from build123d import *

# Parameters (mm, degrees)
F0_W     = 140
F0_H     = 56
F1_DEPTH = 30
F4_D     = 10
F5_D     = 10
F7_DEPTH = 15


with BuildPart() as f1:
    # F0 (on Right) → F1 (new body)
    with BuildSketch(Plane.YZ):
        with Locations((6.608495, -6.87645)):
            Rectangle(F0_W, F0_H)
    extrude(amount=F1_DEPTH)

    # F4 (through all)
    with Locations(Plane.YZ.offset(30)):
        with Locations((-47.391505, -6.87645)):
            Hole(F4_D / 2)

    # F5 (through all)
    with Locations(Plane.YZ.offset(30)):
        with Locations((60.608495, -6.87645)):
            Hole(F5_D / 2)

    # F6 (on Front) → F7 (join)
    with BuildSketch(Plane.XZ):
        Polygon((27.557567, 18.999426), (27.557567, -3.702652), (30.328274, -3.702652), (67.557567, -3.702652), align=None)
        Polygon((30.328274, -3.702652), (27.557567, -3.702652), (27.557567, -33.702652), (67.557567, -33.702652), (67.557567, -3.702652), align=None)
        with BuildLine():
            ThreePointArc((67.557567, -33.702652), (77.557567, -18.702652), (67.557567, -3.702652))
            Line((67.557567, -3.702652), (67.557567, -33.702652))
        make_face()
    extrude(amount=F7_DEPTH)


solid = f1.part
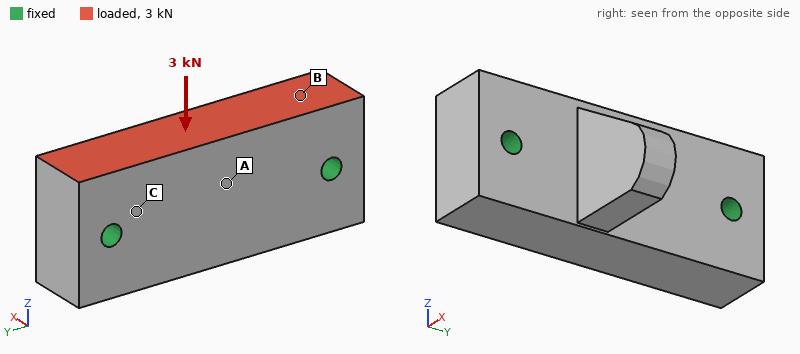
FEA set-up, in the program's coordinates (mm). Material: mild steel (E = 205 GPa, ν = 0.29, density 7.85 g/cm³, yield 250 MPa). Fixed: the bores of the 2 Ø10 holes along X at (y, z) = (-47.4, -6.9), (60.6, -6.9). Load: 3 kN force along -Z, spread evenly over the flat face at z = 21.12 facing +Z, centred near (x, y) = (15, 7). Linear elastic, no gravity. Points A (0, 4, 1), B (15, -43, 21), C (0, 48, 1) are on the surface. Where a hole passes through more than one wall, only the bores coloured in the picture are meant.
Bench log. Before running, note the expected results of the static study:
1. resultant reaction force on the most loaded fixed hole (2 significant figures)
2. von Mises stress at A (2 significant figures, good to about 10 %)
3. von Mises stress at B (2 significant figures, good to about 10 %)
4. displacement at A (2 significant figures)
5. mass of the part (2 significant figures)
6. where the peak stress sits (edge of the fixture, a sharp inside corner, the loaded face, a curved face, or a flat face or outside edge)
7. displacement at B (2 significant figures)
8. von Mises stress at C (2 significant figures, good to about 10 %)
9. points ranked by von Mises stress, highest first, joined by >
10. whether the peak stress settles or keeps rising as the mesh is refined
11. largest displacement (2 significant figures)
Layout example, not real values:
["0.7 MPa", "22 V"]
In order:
["1.5 kN", "0.48 MPa", "0.91 MPa", "0.54 µm", "2.0 kg", "edge of the fixture", "0.26 µm", "1.5 MPa", "C > B > A", "keeps rising", "0.59 µm"]
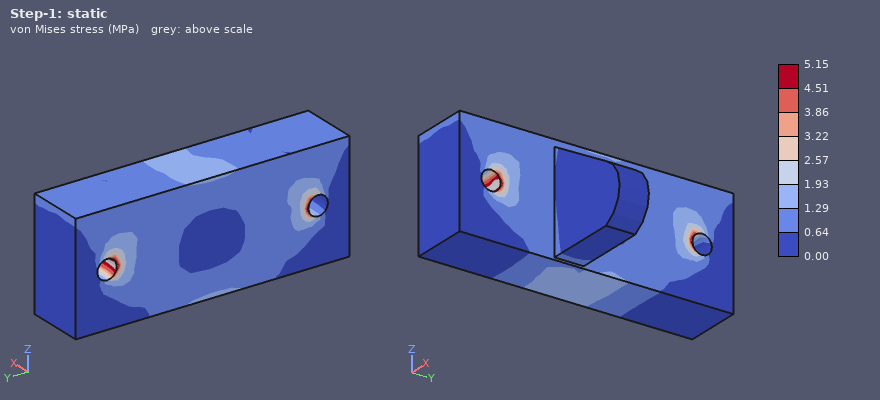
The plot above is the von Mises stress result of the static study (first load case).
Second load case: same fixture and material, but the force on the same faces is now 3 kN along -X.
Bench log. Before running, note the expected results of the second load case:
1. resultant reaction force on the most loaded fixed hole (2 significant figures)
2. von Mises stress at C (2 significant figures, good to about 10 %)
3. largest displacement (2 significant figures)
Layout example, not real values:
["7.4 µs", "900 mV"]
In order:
["1.5 kN", "4.4 MPa", "2.6 µm"]
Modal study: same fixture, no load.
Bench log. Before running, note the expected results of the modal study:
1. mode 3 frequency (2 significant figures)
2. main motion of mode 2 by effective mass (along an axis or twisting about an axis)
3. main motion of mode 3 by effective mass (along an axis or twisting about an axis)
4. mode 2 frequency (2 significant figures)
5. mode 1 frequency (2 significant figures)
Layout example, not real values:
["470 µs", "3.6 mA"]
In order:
["7600 Hz", "along Z", "along X", "6000 Hz", "5200 Hz"]
